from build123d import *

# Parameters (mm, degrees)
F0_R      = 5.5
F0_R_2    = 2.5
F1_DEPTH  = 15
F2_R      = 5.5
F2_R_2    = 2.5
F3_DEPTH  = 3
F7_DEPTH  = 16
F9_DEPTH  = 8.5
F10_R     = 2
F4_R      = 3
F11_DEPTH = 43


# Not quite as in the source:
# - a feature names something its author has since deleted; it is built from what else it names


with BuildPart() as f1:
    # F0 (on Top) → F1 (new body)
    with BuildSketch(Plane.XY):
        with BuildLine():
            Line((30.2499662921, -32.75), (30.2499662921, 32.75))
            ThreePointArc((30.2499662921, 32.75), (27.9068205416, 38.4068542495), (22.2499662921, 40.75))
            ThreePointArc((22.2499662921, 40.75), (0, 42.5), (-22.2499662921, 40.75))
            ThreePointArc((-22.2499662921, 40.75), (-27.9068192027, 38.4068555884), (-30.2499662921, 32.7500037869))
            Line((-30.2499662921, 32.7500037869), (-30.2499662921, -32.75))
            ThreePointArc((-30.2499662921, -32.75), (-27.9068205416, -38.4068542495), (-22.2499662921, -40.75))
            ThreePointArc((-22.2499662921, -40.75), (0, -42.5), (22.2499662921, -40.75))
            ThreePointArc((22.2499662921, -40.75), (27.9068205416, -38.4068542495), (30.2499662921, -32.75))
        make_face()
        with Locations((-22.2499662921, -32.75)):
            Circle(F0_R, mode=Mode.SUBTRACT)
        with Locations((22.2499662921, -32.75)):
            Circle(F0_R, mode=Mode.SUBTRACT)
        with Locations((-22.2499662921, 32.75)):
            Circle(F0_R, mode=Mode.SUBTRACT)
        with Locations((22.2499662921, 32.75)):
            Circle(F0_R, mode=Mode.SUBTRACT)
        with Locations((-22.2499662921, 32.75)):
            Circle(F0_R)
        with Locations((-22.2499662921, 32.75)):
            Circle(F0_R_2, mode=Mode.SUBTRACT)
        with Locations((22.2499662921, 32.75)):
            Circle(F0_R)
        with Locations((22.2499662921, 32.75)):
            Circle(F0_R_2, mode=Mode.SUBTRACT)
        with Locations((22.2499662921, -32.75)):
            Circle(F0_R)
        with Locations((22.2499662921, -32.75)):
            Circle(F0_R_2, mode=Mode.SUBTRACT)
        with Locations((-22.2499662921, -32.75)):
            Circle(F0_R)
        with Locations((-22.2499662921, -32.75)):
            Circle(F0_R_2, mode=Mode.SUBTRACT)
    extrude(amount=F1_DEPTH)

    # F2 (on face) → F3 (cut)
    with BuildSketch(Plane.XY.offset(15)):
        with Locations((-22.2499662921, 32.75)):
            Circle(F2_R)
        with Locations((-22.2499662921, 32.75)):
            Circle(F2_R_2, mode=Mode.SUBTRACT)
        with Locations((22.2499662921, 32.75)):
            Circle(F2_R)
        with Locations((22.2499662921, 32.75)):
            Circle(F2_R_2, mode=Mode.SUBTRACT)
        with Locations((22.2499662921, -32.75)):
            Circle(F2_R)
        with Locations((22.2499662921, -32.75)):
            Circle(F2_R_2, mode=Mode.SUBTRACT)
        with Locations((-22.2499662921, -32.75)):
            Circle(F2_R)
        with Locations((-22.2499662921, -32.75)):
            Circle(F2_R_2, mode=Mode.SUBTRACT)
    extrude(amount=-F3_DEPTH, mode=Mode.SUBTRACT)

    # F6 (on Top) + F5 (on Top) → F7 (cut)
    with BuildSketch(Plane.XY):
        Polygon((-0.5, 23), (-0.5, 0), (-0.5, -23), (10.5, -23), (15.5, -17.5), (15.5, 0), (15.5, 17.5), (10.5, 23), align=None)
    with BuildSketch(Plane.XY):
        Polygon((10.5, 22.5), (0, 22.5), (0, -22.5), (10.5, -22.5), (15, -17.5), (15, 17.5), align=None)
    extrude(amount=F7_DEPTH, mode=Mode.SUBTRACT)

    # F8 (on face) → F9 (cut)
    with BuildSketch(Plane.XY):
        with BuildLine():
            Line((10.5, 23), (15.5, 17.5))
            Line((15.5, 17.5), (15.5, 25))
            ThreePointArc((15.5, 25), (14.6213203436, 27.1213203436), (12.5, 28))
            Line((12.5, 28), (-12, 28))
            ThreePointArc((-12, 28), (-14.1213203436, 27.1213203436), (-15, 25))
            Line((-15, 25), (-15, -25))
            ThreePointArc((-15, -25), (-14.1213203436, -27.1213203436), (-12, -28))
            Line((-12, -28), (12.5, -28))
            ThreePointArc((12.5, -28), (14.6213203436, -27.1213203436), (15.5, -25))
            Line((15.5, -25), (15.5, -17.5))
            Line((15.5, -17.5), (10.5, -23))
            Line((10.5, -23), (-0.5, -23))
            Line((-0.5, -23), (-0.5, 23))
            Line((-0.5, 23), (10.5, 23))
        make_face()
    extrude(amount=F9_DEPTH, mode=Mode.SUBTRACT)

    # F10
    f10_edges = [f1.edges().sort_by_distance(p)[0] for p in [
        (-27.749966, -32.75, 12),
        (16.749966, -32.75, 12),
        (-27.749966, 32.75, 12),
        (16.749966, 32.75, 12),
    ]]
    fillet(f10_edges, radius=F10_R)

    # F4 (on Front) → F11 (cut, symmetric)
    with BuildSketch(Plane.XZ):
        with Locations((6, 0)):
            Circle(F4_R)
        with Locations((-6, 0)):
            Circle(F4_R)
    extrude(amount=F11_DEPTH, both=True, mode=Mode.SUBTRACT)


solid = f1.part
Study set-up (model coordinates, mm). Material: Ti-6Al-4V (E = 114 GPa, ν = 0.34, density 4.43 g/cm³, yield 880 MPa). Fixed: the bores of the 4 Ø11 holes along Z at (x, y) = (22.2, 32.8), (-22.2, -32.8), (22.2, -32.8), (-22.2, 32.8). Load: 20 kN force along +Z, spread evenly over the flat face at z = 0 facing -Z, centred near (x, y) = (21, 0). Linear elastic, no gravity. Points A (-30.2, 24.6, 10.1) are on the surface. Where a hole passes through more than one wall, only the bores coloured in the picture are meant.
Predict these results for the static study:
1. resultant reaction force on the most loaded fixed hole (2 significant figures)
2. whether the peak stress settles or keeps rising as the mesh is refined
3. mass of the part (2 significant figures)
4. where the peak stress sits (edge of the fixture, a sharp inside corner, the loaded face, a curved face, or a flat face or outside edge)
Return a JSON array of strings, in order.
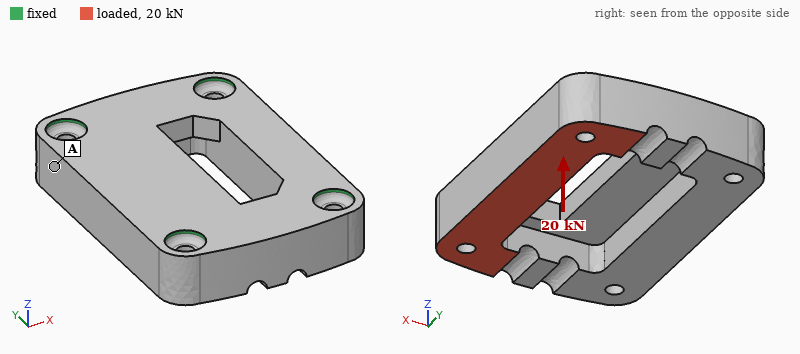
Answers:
["11 kN", "keeps rising", "230 g", "edge of the fixture"]
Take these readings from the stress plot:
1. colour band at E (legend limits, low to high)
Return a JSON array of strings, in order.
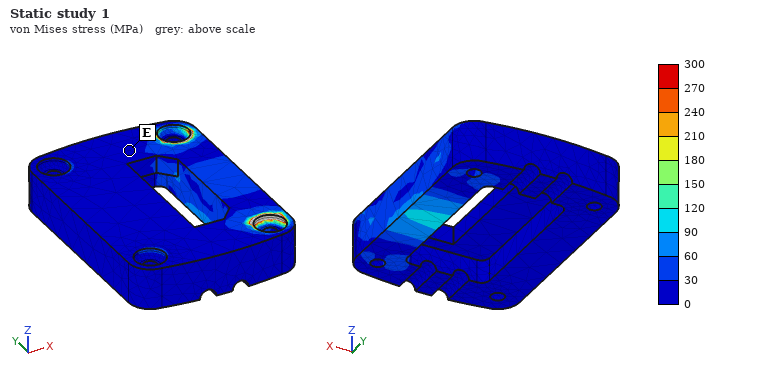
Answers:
["0 to 30 MPa"]
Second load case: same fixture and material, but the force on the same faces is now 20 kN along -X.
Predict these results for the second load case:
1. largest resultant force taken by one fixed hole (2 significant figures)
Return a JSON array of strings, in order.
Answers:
["6.7 kN"]
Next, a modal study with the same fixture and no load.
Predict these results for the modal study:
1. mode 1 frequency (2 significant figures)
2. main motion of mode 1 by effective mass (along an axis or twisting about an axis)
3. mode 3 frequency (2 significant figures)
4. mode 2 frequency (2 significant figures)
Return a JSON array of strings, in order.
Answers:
["10 kHz", "along Z", "13 kHz", "12 kHz"]
